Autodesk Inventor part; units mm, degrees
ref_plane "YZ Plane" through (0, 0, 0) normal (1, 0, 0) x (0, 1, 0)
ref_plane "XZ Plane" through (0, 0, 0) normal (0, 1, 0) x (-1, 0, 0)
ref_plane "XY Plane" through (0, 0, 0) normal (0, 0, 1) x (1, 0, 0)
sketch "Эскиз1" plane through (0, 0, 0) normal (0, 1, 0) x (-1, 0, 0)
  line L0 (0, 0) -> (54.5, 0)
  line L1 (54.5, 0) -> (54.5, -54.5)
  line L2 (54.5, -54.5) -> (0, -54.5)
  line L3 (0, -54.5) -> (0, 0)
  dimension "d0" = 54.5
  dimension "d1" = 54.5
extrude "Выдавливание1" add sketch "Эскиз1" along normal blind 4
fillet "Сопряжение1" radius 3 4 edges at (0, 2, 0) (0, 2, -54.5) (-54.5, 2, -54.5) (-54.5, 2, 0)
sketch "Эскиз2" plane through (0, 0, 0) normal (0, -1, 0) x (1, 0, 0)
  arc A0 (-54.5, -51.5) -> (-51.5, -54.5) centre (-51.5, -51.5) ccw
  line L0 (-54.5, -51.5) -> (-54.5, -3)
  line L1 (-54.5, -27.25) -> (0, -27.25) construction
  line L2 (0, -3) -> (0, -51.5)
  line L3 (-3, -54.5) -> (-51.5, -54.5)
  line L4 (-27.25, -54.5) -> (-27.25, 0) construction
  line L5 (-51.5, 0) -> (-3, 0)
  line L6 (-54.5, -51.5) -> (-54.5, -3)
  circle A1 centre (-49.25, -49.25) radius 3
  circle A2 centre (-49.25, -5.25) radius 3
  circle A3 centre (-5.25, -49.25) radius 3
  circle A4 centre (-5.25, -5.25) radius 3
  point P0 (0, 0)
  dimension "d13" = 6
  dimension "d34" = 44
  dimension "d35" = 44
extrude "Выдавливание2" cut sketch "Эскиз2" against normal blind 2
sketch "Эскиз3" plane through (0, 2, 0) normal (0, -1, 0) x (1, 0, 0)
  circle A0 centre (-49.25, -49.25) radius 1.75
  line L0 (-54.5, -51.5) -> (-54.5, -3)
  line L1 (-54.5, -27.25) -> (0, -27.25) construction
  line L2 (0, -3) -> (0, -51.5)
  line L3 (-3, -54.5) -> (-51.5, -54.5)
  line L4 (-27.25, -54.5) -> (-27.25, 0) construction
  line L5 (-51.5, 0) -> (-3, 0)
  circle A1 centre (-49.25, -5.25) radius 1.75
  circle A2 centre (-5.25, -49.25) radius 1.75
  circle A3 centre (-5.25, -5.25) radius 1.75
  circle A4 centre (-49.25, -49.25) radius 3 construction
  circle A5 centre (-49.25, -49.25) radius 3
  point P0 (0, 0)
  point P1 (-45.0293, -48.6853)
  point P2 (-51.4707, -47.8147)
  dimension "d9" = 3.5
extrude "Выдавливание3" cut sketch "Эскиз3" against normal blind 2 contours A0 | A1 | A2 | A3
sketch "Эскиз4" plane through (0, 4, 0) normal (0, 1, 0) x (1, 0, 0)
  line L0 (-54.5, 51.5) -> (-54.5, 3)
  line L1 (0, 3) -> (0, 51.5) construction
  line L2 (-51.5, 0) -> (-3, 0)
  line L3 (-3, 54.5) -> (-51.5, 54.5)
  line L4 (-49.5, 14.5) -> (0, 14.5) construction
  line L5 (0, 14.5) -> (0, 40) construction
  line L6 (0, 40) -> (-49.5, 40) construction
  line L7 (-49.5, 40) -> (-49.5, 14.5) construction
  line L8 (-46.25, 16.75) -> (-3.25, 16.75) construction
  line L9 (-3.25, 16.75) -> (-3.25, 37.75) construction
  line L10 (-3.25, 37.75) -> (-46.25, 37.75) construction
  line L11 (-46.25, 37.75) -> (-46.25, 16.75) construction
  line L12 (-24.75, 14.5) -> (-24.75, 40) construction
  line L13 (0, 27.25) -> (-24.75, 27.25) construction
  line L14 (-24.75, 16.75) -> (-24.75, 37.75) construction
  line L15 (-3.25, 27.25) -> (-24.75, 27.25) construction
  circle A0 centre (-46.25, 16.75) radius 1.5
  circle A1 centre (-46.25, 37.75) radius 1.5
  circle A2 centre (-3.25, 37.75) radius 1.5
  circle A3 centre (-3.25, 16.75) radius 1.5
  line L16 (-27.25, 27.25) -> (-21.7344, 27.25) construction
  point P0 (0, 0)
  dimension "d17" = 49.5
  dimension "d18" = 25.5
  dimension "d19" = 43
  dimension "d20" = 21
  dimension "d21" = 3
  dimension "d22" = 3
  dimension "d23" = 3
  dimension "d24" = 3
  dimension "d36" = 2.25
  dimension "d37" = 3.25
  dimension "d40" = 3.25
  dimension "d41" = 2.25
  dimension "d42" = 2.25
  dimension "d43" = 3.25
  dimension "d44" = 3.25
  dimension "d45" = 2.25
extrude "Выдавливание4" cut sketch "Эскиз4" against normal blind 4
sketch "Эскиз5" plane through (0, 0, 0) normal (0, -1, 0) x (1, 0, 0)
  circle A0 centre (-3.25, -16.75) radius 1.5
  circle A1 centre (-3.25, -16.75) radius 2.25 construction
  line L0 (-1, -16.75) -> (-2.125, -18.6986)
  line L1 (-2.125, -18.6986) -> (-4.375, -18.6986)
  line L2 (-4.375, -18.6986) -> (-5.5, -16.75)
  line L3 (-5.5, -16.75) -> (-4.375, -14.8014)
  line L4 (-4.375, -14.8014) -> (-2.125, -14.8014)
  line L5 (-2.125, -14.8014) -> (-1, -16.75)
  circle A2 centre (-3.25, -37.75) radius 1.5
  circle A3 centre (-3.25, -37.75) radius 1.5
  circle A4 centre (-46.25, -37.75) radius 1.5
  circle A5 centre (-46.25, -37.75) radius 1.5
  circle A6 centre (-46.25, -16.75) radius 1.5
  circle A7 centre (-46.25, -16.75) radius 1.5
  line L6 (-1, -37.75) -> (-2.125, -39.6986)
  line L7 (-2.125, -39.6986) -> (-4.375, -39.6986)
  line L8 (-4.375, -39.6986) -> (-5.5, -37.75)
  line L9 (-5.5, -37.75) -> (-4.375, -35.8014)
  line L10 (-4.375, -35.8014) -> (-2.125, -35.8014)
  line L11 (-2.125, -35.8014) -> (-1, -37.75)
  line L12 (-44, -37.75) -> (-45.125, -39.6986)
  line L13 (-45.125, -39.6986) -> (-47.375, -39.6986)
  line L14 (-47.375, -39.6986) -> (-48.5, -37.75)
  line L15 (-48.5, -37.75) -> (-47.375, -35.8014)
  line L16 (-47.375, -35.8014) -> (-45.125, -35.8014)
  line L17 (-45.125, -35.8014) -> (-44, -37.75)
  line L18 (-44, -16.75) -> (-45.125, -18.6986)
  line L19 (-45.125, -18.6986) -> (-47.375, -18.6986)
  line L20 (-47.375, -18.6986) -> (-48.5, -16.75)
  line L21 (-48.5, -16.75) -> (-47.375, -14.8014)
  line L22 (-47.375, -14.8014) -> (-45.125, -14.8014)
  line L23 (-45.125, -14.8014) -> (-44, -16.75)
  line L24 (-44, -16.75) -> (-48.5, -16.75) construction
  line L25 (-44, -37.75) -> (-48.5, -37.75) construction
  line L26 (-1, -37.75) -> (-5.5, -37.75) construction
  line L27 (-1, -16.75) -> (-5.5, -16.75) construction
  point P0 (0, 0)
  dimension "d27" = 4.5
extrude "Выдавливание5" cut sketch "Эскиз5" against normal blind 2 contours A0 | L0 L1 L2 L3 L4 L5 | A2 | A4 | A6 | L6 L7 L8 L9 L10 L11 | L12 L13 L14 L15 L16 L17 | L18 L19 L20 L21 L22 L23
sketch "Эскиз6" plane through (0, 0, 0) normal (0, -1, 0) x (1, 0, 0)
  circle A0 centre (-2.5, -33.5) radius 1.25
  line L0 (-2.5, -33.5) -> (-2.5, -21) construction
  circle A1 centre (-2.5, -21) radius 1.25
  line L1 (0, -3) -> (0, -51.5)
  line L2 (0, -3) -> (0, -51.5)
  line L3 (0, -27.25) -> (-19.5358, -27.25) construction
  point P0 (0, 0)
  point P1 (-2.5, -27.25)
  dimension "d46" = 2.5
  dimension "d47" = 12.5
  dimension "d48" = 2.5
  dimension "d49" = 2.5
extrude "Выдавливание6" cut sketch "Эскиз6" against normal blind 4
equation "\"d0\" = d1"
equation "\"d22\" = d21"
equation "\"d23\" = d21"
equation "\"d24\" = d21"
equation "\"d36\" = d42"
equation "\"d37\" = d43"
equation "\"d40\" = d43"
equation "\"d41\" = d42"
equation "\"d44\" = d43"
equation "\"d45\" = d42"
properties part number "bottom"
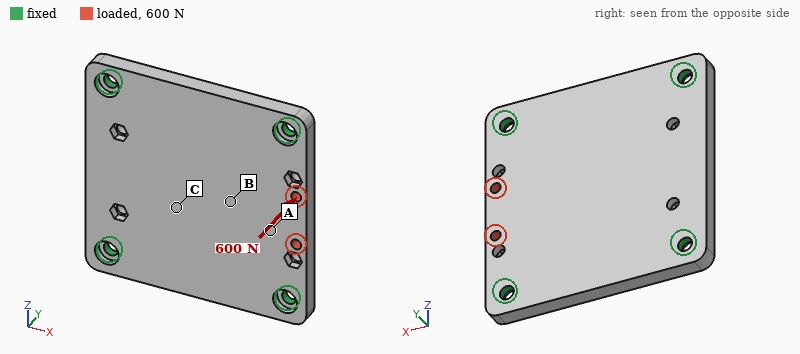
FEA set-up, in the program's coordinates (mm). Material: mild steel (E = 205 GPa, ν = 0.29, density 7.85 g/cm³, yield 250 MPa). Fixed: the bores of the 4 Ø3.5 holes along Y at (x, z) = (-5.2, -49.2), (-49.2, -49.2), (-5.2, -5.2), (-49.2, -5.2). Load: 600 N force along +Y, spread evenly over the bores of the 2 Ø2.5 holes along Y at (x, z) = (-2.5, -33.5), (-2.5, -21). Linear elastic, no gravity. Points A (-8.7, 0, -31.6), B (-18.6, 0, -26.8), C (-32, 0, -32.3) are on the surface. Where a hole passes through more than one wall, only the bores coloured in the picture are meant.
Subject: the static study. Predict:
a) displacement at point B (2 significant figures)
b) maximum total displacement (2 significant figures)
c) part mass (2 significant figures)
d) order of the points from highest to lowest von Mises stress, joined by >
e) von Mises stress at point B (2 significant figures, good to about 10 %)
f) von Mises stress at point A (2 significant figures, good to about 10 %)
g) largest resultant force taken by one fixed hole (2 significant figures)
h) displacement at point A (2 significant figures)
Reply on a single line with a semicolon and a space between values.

8.1 µm; 27 µm; 89 g; A > B > C; 27 MPa; 52 MPa; 460 N; 15 µm
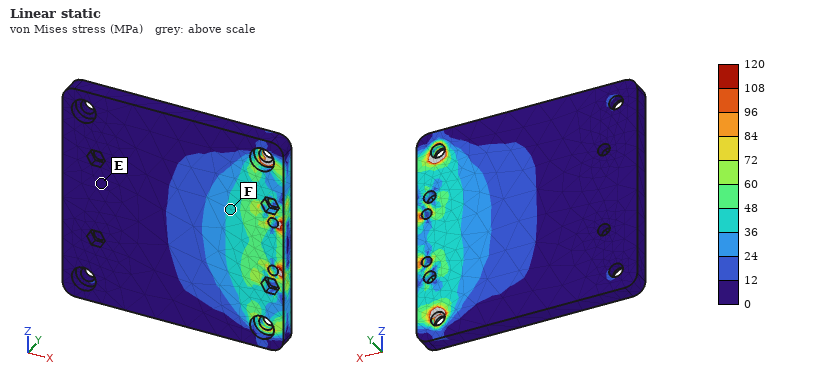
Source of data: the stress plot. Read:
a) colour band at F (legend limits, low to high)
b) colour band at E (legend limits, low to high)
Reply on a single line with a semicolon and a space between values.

36 to 48 MPa; 0 to 12 MPa
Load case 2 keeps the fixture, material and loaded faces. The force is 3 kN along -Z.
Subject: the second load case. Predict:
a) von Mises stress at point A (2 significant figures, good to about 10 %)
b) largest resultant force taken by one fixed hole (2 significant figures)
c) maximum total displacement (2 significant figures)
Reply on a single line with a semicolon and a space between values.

13 MPa; 1.3 kN; 5.4 µm
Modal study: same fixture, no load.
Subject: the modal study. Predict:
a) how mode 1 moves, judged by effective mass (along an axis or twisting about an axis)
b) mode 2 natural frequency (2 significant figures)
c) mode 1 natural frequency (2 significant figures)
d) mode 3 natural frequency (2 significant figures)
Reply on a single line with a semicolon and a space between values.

along Y; 9800 Hz; 5900 Hz; 9800 Hz
